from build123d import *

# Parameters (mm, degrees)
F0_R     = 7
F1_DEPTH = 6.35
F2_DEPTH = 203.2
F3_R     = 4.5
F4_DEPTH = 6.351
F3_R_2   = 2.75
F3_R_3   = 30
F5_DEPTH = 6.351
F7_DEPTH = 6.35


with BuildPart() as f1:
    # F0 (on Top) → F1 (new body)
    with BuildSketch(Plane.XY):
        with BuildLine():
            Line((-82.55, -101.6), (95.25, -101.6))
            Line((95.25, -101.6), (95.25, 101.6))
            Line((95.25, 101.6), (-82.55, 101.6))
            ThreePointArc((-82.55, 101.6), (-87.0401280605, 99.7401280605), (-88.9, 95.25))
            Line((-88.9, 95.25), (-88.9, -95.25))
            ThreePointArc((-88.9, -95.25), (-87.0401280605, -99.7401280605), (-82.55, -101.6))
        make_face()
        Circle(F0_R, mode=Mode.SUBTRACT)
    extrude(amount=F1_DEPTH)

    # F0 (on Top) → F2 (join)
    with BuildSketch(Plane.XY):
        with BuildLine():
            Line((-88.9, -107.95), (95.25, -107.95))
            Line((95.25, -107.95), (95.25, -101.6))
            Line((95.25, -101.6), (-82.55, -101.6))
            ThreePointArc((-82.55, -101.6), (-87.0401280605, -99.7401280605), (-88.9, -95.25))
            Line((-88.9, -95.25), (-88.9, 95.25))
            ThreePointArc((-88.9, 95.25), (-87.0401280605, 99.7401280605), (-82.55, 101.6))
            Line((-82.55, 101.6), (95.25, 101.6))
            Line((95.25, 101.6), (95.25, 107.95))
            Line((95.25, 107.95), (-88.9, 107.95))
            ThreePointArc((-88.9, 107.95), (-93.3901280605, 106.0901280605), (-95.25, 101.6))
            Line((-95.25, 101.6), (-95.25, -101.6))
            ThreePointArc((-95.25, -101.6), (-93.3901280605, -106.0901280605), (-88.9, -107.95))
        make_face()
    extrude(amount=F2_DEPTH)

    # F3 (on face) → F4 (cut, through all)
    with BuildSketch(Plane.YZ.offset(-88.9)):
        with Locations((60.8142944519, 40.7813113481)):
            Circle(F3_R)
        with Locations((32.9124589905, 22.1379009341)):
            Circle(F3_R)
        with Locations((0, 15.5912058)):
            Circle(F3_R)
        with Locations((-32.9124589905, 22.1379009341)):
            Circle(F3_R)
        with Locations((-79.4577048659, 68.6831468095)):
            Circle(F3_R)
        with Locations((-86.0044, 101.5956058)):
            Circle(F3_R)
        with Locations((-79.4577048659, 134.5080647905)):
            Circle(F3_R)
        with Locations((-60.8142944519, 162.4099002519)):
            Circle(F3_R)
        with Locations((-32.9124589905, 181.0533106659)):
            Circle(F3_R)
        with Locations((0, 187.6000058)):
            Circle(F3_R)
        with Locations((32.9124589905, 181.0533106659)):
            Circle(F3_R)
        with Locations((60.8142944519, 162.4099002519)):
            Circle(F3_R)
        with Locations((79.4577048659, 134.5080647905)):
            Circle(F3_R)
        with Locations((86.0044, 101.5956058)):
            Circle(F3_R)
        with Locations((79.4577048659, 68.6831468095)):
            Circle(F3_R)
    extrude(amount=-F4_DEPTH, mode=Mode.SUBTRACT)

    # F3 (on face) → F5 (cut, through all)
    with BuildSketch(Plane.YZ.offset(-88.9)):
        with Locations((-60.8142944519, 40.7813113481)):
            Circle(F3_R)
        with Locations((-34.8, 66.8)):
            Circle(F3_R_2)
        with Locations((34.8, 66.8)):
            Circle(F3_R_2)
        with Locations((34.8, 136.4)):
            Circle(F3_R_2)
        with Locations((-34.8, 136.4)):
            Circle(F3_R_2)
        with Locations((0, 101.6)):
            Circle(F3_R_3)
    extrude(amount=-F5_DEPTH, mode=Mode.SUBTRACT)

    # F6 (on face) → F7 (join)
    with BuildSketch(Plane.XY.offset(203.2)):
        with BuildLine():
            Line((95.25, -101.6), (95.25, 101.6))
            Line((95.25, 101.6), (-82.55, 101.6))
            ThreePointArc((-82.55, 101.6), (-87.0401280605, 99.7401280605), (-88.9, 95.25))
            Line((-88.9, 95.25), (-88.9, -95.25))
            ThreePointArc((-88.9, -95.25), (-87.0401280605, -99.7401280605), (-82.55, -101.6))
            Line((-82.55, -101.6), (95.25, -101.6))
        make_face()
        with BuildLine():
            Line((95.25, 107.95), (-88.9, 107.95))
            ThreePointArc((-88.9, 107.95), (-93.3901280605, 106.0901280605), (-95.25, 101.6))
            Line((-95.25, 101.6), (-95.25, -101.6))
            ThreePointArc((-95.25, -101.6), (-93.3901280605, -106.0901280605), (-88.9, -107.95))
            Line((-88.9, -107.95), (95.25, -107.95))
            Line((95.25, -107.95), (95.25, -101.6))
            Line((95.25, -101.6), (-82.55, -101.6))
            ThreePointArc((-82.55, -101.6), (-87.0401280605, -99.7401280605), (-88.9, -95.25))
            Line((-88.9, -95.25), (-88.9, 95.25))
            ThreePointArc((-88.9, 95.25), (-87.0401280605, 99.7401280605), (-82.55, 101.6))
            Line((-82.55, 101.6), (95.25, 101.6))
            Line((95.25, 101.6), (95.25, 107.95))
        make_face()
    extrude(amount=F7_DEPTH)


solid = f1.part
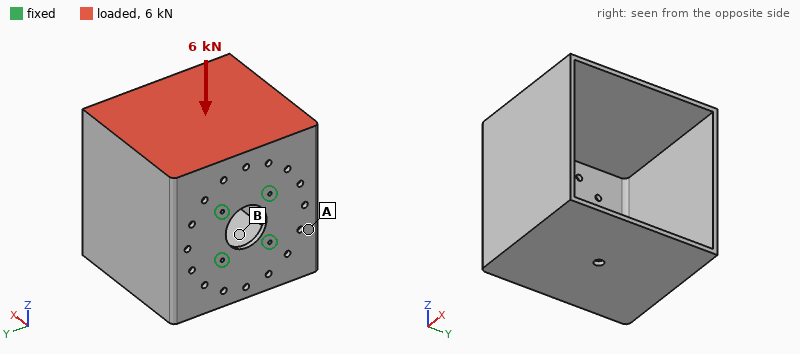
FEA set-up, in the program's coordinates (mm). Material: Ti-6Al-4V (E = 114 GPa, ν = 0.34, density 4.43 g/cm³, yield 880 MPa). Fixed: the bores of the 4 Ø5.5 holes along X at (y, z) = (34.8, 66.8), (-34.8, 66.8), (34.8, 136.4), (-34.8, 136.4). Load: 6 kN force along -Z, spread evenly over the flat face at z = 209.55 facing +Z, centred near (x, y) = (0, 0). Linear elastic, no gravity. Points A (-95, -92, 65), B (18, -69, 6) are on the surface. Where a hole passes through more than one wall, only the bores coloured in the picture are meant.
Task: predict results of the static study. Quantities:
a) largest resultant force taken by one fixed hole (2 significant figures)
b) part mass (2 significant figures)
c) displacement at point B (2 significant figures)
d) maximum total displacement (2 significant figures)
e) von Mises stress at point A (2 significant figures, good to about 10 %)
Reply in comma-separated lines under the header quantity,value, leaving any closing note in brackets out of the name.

quantity,value
largest resultant force taken by one fixed hole,3.4 kN
part mass,5.4 kg
displacement at point B,0.75 mm
maximum total displacement,1.7 mm
von Mises stress at point A,23 MPa
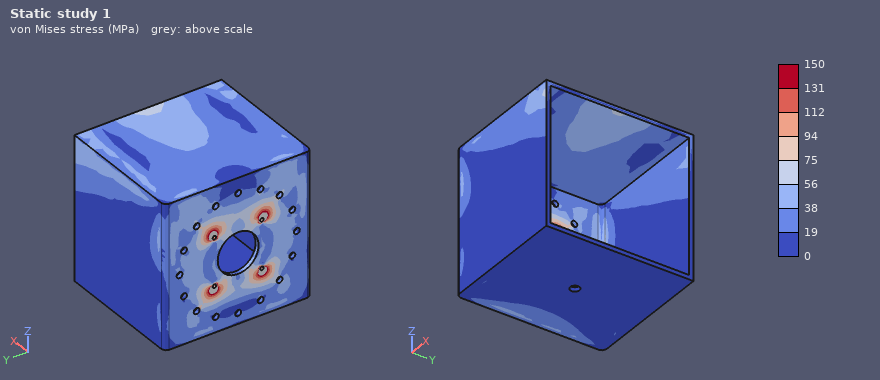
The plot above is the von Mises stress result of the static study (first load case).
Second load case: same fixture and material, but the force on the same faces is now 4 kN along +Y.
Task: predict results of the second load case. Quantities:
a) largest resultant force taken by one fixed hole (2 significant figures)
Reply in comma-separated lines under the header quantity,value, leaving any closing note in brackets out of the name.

quantity,value
largest resultant force taken by one fixed hole,3.9 kN
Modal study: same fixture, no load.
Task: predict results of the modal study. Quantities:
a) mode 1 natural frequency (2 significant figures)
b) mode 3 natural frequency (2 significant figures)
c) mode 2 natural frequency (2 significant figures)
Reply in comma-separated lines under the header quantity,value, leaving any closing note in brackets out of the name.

quantity,value
mode 1 natural frequency,180 Hz
mode 3 natural frequency,260 Hz
mode 2 natural frequency,180 Hz
